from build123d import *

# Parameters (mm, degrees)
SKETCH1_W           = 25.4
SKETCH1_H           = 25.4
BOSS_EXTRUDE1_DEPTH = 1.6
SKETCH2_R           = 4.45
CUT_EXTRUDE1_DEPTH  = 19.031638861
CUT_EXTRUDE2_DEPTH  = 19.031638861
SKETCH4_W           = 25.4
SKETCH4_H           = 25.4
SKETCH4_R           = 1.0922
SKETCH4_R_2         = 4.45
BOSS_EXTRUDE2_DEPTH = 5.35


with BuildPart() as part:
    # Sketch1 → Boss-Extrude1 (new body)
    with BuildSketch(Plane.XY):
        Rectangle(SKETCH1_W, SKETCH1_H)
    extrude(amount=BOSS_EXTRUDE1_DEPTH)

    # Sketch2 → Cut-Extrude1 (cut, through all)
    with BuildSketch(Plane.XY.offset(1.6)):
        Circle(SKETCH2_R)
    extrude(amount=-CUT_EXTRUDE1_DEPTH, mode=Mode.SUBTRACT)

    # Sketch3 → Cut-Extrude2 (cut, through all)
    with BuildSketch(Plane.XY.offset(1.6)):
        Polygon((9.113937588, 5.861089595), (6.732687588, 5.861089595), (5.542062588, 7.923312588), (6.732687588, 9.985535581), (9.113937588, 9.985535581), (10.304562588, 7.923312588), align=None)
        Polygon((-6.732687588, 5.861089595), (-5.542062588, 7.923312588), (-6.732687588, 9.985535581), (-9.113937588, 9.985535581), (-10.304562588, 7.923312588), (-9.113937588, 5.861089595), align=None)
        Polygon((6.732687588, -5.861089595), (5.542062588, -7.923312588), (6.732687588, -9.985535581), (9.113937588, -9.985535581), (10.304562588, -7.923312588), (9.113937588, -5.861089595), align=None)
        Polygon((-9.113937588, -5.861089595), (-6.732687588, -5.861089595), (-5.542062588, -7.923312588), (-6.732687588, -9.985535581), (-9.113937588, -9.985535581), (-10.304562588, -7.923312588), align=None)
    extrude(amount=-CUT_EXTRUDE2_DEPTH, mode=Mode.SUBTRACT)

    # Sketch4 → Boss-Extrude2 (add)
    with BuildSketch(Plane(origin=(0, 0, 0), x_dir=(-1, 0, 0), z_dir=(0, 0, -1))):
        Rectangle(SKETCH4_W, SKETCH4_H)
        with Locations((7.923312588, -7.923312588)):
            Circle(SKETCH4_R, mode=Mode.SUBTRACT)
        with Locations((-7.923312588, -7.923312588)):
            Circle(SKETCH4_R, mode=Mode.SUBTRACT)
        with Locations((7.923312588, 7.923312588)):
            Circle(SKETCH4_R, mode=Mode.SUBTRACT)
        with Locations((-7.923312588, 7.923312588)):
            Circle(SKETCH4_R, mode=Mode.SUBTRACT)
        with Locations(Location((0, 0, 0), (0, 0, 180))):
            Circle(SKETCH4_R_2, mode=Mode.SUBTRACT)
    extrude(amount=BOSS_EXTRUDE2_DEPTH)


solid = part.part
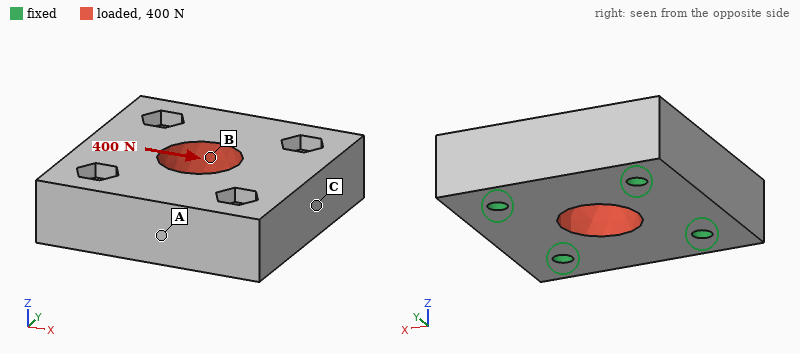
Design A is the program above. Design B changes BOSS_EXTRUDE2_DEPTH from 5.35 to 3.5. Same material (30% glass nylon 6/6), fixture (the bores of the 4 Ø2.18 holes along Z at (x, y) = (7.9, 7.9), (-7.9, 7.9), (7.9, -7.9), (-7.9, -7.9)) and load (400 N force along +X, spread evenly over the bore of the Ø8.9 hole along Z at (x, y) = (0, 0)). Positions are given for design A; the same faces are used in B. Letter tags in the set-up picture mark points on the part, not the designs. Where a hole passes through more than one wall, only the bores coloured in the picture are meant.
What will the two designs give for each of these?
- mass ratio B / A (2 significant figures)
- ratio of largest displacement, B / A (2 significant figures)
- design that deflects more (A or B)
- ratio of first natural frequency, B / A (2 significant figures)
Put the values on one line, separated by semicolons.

0.73; 1.4; B; 0.84
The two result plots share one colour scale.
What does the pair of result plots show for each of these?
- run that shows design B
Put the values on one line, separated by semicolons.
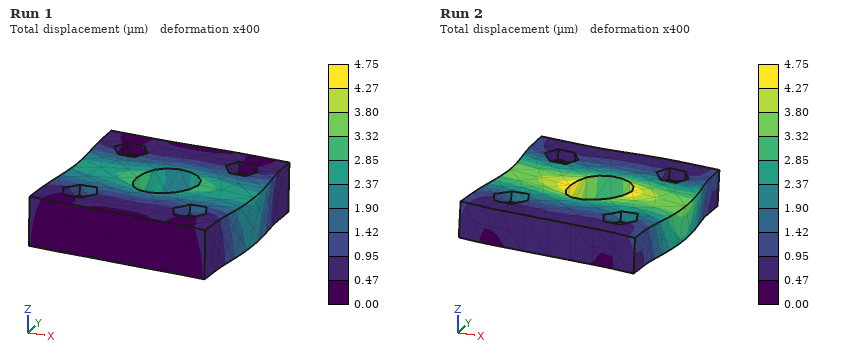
Run 2
